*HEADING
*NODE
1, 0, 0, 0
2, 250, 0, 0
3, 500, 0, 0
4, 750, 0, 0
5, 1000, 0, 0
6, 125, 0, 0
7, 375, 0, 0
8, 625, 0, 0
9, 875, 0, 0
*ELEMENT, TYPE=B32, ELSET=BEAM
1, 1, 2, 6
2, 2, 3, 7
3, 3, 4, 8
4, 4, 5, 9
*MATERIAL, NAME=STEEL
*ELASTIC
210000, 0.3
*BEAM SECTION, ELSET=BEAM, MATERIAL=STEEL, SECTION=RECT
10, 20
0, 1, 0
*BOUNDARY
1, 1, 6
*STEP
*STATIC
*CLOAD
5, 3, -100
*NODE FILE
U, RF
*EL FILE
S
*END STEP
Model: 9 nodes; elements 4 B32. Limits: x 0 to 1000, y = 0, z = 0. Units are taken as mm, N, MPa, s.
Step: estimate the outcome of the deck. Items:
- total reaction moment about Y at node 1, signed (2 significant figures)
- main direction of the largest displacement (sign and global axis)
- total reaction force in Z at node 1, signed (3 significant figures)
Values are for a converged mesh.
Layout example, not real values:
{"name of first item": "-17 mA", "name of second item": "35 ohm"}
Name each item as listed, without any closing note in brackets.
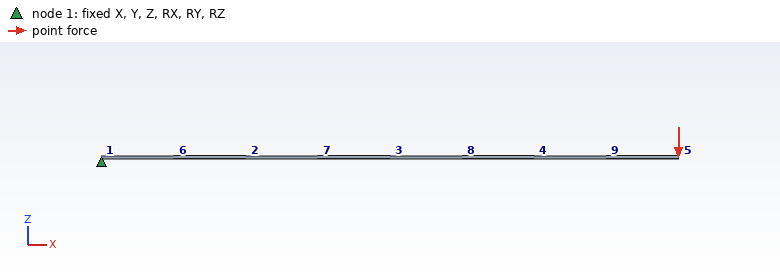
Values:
{"total reaction moment about Y at node 1, signed": "-100000 N·mm", "main direction of the largest displacement": "-Z", "total reaction force in Z at node 1, signed": "100 N"}
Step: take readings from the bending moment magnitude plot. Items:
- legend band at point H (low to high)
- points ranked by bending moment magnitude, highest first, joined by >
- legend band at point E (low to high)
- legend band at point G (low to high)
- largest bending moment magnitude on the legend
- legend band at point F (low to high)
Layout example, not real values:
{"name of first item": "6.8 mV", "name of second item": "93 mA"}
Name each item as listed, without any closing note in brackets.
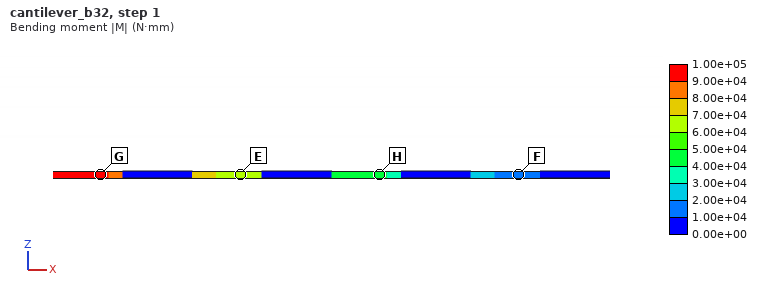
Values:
{"legend band at point H": "4.00e+04 to 5.00e+04 N·mm", "points ranked by bending moment magnitude, highest first, joined by >": "G > E > H > F", "legend band at point E": "6.00e+04 to 7.00e+04 N·mm", "legend band at point G": "9.00e+04 to 1.00e+05 N·mm", "largest bending moment magnitude on the legend": "1.00e+05 N·mm", "legend band at point F": "1.00e+04 to 2.00e+04 N·mm"}
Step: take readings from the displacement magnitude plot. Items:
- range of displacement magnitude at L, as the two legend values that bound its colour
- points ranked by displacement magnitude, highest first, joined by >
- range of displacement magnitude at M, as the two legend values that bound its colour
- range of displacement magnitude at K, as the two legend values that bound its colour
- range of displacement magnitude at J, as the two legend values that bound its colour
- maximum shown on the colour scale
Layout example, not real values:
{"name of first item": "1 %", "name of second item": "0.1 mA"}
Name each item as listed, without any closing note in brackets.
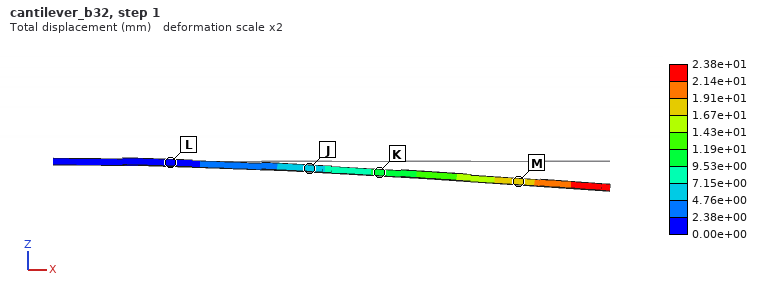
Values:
{"range of displacement magnitude at L, as the two legend values that bound its colour": "0.00e+00 to 2.38e+00 mm", "points ranked by displacement magnitude, highest first, joined by >": "M > K > J > L", "range of displacement magnitude at M, as the two legend values that bound its colour": "1.67e+01 to 1.91e+01 mm", "range of displacement magnitude at K, as the two legend values that bound its colour": "9.53e+00 to 1.19e+01 mm", "range of displacement magnitude at J, as the two legend values that bound its colour": "4.76e+00 to 7.15e+00 mm", "maximum shown on the colour scale": "2.38e+01 mm"}
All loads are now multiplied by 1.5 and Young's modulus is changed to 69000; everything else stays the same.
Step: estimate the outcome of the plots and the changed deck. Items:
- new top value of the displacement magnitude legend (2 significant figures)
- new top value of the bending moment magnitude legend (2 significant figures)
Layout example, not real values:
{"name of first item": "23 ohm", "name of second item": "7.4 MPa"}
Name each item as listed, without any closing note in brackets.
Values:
{"new top value of the displacement magnitude legend": "110 mm", "new top value of the bending moment magnitude legend": "1.5e+05 N·mm"}
